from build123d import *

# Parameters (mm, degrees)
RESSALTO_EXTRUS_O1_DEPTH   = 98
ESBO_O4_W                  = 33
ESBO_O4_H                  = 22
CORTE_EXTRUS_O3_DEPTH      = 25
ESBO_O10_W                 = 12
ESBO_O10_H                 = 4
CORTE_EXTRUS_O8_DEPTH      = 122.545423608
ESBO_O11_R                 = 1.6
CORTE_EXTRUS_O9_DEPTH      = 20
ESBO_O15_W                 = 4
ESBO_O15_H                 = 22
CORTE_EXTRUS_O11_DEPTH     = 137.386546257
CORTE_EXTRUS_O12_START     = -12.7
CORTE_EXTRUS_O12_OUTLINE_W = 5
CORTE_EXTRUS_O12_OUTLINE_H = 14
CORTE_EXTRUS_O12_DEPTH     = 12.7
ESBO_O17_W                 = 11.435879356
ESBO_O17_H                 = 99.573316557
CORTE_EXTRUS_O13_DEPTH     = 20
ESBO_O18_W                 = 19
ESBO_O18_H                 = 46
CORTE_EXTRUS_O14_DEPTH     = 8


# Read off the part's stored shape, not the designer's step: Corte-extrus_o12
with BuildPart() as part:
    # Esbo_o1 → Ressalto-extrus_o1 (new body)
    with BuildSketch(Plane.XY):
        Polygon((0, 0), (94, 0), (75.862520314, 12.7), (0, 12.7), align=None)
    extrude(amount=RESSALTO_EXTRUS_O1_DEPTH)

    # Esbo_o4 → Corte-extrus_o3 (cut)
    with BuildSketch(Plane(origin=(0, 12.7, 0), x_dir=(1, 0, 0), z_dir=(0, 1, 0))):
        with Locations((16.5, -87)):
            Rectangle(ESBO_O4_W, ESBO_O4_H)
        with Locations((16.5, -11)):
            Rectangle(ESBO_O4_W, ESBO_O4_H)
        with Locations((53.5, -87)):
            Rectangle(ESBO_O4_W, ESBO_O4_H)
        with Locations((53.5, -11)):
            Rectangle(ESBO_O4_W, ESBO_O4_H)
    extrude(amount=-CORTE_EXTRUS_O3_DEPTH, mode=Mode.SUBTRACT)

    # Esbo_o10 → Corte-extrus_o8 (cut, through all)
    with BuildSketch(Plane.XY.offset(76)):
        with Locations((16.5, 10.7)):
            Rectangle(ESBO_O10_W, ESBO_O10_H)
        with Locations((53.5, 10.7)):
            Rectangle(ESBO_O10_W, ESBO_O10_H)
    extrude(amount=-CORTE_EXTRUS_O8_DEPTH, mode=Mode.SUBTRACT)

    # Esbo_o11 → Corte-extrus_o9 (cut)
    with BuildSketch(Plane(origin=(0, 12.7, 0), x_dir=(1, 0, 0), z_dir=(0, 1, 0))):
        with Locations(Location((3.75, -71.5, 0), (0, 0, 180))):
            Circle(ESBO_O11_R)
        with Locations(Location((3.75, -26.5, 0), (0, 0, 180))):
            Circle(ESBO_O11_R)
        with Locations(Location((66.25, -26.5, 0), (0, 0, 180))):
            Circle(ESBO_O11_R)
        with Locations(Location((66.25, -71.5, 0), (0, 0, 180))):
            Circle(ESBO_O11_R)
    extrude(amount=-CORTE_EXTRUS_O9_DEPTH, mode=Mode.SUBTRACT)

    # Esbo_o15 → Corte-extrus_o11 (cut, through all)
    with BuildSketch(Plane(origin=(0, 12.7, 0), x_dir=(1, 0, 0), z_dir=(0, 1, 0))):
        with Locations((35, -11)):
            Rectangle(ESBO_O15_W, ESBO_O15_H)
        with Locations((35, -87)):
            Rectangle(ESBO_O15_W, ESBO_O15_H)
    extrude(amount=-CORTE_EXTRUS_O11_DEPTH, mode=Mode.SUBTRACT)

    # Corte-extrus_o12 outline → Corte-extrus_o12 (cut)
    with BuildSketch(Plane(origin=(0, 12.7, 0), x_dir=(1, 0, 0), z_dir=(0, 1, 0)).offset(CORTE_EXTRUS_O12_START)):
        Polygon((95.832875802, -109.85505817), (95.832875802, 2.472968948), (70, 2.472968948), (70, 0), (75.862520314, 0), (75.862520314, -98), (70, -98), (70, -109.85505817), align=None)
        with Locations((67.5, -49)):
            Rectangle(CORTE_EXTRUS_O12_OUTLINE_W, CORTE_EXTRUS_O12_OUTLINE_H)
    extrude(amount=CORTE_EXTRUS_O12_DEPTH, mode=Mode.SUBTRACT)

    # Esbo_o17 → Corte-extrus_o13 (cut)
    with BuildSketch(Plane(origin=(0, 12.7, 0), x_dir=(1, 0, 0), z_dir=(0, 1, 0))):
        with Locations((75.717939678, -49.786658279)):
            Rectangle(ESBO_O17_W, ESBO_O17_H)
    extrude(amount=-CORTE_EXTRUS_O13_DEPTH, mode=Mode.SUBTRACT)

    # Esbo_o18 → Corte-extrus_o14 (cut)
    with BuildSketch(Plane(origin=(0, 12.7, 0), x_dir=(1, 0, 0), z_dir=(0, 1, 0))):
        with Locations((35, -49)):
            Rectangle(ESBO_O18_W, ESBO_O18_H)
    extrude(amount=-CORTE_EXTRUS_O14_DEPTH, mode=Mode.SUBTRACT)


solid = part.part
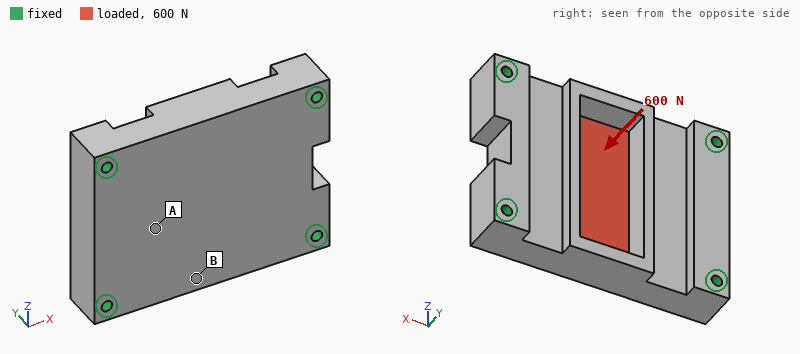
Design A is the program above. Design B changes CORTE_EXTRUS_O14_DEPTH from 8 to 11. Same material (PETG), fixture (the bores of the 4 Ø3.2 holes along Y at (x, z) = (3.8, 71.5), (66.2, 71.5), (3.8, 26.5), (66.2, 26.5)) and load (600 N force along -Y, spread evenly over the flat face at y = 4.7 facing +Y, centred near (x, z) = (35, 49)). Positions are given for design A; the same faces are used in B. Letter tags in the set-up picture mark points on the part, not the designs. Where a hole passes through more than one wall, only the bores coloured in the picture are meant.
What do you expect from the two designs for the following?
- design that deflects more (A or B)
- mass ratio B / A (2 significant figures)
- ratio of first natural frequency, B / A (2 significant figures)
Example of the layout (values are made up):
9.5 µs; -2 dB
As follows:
B; 0.92; 1.1
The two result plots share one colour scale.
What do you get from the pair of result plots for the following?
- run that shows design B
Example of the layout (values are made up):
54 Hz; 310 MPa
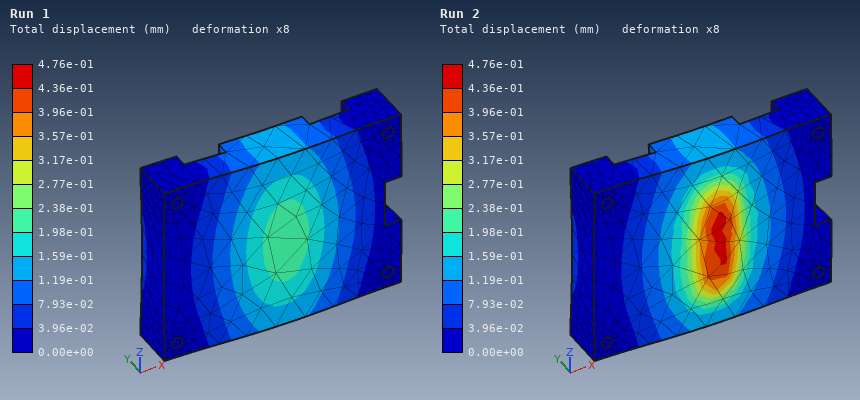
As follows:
Run 2
